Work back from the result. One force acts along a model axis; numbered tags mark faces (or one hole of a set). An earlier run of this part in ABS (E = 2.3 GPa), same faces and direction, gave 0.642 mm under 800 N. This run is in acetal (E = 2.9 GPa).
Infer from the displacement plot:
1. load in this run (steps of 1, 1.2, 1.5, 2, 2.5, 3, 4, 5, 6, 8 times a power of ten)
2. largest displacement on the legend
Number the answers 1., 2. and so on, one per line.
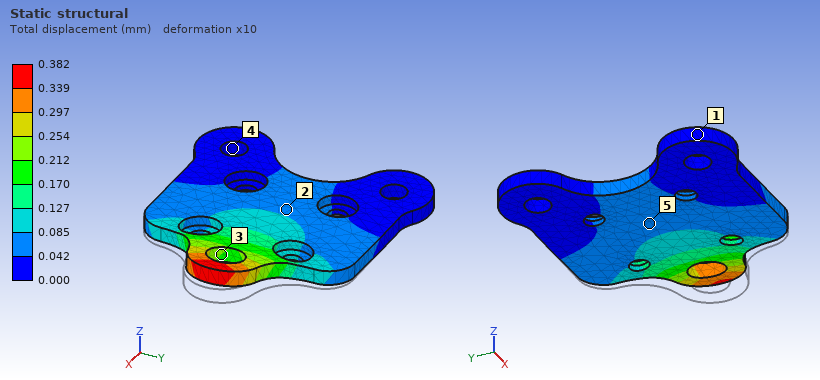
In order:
1. 600 N
2. 0.382 mm
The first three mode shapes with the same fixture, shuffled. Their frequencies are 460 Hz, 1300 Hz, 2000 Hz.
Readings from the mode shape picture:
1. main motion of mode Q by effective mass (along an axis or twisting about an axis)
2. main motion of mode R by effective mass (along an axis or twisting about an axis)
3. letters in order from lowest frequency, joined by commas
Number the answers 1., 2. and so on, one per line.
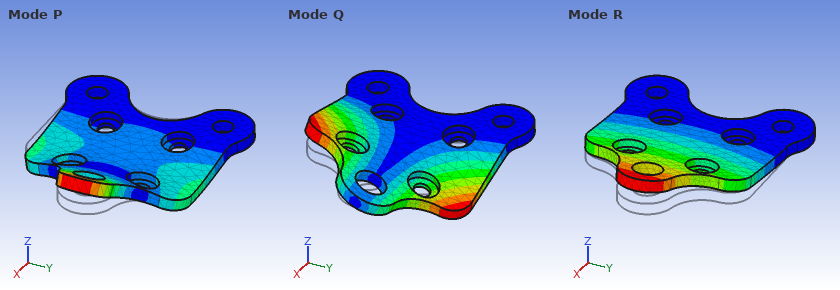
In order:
1. twisting about X
2. along Z
3. R, Q, P
